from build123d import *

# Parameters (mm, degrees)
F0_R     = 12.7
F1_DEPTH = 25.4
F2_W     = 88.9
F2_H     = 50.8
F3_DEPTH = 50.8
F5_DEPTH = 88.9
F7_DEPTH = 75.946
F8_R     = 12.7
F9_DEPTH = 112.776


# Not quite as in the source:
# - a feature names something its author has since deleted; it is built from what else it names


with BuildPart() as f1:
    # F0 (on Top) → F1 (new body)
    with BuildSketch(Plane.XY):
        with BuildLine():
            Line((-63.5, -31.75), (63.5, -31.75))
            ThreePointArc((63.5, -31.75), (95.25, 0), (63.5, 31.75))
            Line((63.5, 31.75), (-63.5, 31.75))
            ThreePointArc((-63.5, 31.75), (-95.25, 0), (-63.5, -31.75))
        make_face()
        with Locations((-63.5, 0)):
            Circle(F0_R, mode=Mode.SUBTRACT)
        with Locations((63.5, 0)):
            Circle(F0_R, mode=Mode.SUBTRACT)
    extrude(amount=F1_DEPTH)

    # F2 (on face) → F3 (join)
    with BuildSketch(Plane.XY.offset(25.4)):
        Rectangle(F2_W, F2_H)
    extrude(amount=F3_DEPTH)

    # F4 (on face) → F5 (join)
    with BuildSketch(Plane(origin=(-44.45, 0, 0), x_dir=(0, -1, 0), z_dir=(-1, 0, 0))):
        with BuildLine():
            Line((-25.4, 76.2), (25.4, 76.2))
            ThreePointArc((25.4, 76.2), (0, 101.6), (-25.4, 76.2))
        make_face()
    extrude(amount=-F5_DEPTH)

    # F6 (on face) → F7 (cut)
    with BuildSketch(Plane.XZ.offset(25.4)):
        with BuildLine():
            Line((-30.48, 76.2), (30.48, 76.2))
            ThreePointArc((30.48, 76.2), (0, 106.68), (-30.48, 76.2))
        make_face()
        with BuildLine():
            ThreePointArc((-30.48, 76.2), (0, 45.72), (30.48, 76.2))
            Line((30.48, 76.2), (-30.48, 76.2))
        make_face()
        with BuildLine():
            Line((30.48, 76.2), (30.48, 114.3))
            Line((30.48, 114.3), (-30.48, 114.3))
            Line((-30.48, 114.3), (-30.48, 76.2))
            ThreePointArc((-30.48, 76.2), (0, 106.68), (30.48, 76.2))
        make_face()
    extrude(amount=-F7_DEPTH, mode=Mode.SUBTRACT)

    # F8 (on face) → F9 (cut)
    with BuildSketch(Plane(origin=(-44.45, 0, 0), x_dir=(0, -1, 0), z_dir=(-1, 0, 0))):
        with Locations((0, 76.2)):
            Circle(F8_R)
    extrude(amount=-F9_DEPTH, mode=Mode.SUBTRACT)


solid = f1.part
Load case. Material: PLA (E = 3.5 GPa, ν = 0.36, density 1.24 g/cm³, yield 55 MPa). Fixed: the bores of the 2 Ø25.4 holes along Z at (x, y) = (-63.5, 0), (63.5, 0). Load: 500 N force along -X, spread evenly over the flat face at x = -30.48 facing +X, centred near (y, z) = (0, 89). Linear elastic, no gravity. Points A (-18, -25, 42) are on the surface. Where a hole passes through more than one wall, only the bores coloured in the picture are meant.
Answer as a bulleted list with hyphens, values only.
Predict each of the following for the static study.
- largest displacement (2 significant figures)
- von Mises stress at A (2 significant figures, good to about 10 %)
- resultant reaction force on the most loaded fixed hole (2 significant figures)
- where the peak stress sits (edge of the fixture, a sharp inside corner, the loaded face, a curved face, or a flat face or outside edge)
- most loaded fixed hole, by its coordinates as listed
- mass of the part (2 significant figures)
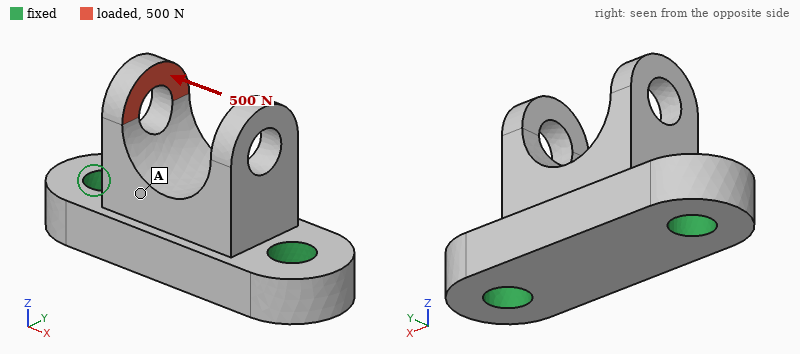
- 0.47 mm
- 1.4 MPa
- 540 N
- a curved face
- (63.5, 0)
- 530 g
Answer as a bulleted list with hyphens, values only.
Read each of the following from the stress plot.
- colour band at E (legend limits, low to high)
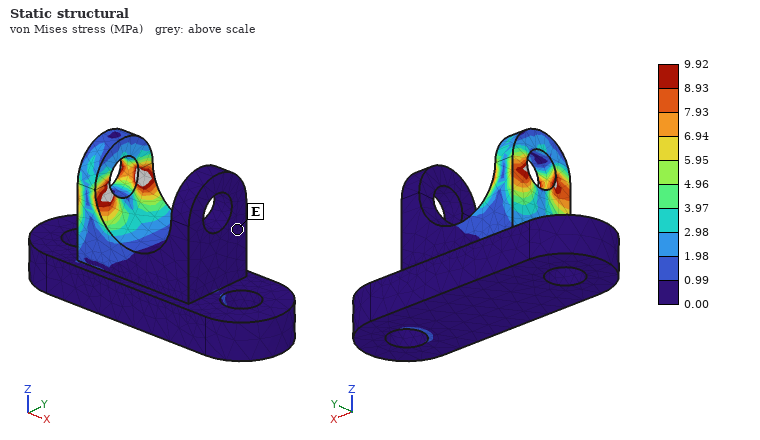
- 0.00 to 0.99 MPa
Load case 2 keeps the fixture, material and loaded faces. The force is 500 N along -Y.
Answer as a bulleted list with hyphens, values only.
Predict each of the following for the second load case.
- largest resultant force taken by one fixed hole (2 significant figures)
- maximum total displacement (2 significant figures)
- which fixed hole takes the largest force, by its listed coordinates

- 370 N
- 0.27 mm
- (-63.5, 0)
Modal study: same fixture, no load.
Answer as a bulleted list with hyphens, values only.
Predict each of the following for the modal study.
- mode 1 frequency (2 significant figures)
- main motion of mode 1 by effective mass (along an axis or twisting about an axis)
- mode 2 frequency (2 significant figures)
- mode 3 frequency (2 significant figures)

- 1300 Hz
- along Y
- 1600 Hz
- 1700 Hz
